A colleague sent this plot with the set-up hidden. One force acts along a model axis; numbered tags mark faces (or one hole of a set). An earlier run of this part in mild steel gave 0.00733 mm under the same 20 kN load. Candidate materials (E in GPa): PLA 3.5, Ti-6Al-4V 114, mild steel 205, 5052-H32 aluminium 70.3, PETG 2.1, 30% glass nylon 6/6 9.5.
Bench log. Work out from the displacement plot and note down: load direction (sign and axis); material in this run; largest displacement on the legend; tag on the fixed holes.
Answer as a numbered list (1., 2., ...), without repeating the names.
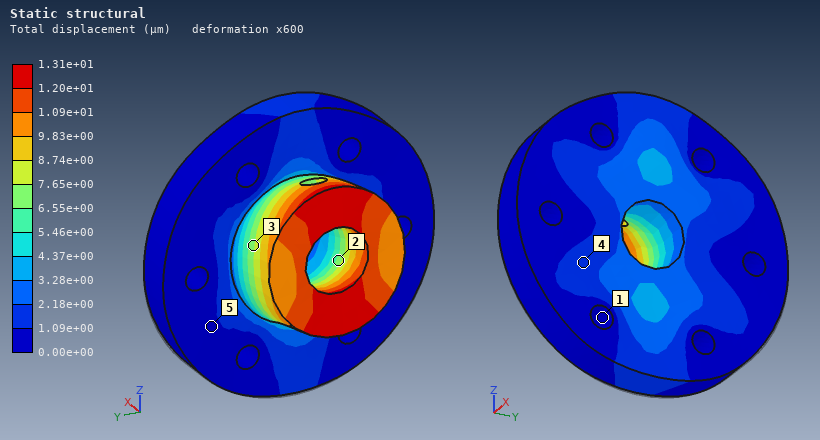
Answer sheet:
1. +Z
2. Ti-6Al-4V
3. 1.31e+01 µm
4. 1
